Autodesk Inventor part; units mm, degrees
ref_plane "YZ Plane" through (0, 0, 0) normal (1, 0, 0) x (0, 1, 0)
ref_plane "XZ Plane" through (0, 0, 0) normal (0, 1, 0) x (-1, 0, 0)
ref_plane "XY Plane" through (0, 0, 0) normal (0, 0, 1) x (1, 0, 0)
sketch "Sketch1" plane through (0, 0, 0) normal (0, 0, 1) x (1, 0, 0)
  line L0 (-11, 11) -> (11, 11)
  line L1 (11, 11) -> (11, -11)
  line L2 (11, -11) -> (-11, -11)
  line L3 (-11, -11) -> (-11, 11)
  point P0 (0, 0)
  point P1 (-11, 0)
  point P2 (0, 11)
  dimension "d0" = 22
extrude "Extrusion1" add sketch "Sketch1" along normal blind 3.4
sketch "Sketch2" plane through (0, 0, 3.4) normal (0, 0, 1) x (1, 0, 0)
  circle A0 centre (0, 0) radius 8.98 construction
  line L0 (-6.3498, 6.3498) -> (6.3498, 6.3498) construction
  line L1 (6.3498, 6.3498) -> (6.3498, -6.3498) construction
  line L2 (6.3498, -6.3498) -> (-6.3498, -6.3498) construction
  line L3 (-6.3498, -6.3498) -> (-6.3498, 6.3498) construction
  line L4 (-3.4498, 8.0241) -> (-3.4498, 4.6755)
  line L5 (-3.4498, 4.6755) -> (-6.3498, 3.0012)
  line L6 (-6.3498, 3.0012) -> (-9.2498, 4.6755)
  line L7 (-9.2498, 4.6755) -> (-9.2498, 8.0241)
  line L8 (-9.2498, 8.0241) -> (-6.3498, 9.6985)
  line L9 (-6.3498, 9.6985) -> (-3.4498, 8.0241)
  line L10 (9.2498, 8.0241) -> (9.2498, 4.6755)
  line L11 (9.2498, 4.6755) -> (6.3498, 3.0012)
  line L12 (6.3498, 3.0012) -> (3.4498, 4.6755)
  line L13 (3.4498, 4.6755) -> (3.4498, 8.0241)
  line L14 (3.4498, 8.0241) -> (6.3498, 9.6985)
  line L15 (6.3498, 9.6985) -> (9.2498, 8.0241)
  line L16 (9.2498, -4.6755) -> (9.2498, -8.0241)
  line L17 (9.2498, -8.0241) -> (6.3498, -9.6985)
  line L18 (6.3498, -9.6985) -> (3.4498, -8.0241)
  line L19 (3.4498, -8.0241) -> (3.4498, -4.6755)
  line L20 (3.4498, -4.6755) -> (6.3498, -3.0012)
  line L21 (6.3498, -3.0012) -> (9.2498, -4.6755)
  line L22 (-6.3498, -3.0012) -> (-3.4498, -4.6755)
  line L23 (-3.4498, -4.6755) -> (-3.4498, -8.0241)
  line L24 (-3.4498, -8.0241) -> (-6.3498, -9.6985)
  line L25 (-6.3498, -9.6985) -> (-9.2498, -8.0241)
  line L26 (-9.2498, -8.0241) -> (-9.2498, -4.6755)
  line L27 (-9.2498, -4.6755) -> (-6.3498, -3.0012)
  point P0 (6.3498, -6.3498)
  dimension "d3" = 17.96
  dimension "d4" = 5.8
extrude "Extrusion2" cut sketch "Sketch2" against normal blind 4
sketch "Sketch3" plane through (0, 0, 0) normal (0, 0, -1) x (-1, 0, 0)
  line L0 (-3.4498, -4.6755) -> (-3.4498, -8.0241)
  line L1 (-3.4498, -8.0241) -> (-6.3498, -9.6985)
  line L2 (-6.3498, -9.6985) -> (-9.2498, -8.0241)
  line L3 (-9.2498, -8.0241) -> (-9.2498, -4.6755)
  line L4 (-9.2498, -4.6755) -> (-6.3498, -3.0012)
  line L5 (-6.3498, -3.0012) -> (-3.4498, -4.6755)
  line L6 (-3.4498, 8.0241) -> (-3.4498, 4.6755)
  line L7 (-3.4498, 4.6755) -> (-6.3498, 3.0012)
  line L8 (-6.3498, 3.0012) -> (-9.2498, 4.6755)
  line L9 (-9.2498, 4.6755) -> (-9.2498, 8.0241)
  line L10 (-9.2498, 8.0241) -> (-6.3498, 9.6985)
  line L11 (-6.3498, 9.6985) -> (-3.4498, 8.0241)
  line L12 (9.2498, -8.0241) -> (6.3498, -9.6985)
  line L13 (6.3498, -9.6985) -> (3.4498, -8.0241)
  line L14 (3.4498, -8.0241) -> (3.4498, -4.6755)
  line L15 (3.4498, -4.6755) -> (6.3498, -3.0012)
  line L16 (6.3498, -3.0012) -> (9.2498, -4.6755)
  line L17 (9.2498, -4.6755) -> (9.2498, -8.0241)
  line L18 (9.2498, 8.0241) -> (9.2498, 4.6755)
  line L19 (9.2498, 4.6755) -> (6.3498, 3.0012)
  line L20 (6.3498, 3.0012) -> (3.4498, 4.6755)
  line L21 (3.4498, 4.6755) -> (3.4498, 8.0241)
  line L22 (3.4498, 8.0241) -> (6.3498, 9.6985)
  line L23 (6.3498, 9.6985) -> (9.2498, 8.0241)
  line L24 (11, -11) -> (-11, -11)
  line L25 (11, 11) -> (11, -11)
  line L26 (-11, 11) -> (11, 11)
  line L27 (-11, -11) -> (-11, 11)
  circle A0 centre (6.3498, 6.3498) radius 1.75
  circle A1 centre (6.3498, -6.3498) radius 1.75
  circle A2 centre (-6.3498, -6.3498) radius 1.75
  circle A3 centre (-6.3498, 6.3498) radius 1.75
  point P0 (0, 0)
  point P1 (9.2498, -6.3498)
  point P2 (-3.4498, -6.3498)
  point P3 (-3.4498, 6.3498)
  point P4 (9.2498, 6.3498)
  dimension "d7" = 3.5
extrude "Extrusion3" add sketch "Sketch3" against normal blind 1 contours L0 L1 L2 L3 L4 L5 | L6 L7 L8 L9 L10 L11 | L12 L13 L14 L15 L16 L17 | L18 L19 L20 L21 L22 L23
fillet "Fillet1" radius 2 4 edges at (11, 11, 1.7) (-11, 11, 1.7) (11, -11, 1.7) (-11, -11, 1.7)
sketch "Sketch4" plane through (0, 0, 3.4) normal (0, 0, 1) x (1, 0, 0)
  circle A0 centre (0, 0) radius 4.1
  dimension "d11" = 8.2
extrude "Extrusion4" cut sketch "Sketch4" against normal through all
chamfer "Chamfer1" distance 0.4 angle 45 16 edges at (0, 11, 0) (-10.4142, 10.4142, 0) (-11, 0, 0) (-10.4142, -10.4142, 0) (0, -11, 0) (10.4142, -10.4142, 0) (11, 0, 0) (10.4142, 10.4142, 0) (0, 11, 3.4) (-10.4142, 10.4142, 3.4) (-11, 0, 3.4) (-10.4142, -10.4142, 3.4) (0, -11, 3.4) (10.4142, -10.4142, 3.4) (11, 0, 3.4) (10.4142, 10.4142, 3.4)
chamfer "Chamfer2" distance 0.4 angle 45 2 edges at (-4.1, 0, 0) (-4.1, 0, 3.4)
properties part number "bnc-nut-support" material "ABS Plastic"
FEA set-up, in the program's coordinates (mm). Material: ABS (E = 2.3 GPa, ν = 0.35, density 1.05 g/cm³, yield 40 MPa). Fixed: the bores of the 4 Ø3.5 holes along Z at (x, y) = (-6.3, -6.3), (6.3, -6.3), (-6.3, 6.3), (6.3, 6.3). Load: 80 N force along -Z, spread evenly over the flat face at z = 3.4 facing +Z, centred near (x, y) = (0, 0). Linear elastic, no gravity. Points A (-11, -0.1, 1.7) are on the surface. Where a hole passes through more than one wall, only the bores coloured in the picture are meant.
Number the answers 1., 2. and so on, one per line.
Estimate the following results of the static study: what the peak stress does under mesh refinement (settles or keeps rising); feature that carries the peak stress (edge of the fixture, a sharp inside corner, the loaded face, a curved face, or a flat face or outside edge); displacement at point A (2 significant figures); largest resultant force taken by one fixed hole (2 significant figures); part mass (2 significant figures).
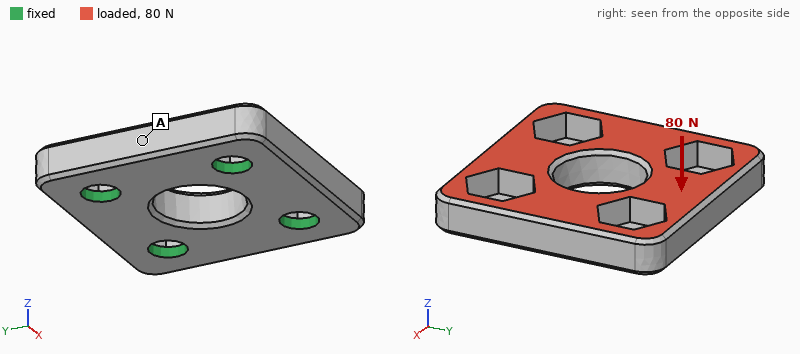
1. keeps rising
2. edge of the fixture
3. 9.3 µm
4. 20 N
5. 1.2 g
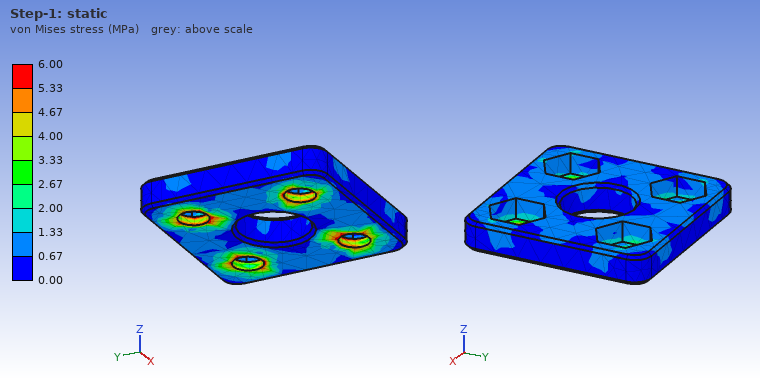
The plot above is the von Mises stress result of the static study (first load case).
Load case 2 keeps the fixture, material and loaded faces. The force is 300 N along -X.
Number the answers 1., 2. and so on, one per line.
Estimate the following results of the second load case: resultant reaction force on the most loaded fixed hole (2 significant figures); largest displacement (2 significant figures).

1. 81 N
2. 60 µm
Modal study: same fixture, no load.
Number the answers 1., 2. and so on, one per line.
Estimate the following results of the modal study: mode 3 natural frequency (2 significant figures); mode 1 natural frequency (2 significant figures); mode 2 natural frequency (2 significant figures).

1. 14 kHz
2. 12 kHz
3. 14 kHz
